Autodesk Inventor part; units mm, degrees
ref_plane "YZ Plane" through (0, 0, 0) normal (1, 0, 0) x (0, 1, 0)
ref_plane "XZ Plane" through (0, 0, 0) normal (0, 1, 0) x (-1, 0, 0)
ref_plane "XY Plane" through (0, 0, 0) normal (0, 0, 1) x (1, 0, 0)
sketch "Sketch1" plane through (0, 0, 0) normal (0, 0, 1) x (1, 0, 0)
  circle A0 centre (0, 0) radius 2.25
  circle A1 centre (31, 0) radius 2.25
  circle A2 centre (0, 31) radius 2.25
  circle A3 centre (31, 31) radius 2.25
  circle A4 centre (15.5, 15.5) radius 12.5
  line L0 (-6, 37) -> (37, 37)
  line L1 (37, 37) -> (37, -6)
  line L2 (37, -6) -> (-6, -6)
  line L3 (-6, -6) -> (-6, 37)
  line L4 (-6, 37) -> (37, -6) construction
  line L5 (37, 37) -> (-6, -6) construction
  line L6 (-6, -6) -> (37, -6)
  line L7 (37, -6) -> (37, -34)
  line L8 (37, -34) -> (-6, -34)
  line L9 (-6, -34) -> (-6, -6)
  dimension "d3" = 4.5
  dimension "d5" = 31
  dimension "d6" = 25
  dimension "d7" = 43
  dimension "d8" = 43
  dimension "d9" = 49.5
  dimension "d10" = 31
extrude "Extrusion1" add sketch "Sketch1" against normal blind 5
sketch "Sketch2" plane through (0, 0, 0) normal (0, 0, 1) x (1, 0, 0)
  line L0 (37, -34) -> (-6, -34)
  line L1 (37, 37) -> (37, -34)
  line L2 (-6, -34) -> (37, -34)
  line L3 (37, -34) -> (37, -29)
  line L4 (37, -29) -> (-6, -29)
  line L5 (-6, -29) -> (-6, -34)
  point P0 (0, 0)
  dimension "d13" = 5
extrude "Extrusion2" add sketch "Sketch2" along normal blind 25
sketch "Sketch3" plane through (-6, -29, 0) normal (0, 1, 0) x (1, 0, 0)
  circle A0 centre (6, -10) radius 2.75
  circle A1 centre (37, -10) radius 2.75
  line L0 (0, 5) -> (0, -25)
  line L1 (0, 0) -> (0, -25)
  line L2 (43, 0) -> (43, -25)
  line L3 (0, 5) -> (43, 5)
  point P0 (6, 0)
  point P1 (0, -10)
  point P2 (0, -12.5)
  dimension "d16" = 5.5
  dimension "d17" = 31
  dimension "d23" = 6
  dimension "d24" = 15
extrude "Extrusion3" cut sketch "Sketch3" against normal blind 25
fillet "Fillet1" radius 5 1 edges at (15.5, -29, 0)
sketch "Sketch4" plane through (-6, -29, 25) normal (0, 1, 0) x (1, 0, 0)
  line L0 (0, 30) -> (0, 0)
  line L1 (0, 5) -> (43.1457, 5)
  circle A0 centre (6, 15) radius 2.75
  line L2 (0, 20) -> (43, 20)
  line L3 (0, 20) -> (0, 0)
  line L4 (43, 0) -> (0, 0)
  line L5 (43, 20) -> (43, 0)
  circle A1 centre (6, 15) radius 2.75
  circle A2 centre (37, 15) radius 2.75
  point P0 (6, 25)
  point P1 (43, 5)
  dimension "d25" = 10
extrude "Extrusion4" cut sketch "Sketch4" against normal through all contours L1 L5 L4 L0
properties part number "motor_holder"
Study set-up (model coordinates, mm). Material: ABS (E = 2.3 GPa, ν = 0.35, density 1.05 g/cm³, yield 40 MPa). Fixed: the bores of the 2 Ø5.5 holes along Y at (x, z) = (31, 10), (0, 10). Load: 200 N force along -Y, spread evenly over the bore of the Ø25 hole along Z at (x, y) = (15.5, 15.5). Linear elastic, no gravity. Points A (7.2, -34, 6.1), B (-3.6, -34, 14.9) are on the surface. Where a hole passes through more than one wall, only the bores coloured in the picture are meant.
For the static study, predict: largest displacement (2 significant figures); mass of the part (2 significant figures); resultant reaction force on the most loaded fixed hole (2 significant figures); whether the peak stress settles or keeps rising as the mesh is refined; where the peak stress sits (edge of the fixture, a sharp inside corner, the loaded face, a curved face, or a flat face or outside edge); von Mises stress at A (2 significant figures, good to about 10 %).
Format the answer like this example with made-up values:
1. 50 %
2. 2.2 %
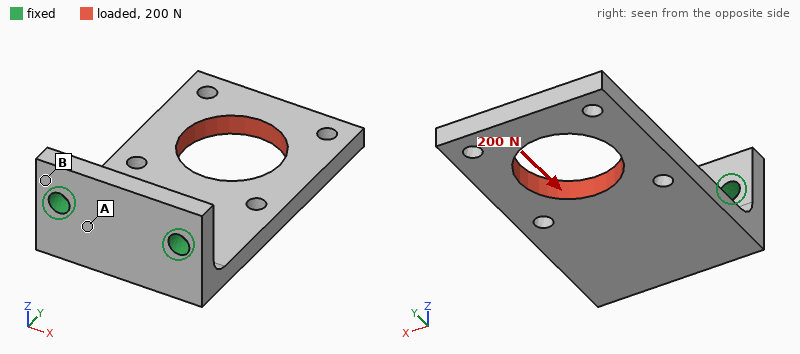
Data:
1. 0.91 mm
2. 18 g
3. 100 N
4. keeps rising
5. edge of the fixture
6. 5.2 MPa
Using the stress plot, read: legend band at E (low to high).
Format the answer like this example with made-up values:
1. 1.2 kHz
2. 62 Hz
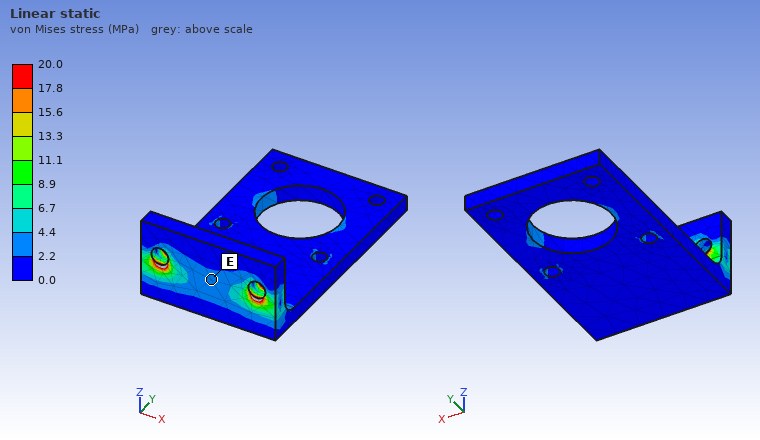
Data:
1. 2.2 to 4.4 MPa
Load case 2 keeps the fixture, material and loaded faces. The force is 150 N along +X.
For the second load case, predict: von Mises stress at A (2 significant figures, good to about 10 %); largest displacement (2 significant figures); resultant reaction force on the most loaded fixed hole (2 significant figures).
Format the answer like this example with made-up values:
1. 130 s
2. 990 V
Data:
1. 4.8 MPa
2. 0.92 mm
3. 230 N
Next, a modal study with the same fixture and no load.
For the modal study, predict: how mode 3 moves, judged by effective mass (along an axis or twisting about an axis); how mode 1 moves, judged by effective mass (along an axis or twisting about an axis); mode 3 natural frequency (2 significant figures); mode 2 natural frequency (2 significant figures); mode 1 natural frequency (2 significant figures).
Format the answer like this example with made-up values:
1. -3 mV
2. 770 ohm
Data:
1. along X
2. along Z
3. 960 Hz
4. 740 Hz
5. 250 Hz
